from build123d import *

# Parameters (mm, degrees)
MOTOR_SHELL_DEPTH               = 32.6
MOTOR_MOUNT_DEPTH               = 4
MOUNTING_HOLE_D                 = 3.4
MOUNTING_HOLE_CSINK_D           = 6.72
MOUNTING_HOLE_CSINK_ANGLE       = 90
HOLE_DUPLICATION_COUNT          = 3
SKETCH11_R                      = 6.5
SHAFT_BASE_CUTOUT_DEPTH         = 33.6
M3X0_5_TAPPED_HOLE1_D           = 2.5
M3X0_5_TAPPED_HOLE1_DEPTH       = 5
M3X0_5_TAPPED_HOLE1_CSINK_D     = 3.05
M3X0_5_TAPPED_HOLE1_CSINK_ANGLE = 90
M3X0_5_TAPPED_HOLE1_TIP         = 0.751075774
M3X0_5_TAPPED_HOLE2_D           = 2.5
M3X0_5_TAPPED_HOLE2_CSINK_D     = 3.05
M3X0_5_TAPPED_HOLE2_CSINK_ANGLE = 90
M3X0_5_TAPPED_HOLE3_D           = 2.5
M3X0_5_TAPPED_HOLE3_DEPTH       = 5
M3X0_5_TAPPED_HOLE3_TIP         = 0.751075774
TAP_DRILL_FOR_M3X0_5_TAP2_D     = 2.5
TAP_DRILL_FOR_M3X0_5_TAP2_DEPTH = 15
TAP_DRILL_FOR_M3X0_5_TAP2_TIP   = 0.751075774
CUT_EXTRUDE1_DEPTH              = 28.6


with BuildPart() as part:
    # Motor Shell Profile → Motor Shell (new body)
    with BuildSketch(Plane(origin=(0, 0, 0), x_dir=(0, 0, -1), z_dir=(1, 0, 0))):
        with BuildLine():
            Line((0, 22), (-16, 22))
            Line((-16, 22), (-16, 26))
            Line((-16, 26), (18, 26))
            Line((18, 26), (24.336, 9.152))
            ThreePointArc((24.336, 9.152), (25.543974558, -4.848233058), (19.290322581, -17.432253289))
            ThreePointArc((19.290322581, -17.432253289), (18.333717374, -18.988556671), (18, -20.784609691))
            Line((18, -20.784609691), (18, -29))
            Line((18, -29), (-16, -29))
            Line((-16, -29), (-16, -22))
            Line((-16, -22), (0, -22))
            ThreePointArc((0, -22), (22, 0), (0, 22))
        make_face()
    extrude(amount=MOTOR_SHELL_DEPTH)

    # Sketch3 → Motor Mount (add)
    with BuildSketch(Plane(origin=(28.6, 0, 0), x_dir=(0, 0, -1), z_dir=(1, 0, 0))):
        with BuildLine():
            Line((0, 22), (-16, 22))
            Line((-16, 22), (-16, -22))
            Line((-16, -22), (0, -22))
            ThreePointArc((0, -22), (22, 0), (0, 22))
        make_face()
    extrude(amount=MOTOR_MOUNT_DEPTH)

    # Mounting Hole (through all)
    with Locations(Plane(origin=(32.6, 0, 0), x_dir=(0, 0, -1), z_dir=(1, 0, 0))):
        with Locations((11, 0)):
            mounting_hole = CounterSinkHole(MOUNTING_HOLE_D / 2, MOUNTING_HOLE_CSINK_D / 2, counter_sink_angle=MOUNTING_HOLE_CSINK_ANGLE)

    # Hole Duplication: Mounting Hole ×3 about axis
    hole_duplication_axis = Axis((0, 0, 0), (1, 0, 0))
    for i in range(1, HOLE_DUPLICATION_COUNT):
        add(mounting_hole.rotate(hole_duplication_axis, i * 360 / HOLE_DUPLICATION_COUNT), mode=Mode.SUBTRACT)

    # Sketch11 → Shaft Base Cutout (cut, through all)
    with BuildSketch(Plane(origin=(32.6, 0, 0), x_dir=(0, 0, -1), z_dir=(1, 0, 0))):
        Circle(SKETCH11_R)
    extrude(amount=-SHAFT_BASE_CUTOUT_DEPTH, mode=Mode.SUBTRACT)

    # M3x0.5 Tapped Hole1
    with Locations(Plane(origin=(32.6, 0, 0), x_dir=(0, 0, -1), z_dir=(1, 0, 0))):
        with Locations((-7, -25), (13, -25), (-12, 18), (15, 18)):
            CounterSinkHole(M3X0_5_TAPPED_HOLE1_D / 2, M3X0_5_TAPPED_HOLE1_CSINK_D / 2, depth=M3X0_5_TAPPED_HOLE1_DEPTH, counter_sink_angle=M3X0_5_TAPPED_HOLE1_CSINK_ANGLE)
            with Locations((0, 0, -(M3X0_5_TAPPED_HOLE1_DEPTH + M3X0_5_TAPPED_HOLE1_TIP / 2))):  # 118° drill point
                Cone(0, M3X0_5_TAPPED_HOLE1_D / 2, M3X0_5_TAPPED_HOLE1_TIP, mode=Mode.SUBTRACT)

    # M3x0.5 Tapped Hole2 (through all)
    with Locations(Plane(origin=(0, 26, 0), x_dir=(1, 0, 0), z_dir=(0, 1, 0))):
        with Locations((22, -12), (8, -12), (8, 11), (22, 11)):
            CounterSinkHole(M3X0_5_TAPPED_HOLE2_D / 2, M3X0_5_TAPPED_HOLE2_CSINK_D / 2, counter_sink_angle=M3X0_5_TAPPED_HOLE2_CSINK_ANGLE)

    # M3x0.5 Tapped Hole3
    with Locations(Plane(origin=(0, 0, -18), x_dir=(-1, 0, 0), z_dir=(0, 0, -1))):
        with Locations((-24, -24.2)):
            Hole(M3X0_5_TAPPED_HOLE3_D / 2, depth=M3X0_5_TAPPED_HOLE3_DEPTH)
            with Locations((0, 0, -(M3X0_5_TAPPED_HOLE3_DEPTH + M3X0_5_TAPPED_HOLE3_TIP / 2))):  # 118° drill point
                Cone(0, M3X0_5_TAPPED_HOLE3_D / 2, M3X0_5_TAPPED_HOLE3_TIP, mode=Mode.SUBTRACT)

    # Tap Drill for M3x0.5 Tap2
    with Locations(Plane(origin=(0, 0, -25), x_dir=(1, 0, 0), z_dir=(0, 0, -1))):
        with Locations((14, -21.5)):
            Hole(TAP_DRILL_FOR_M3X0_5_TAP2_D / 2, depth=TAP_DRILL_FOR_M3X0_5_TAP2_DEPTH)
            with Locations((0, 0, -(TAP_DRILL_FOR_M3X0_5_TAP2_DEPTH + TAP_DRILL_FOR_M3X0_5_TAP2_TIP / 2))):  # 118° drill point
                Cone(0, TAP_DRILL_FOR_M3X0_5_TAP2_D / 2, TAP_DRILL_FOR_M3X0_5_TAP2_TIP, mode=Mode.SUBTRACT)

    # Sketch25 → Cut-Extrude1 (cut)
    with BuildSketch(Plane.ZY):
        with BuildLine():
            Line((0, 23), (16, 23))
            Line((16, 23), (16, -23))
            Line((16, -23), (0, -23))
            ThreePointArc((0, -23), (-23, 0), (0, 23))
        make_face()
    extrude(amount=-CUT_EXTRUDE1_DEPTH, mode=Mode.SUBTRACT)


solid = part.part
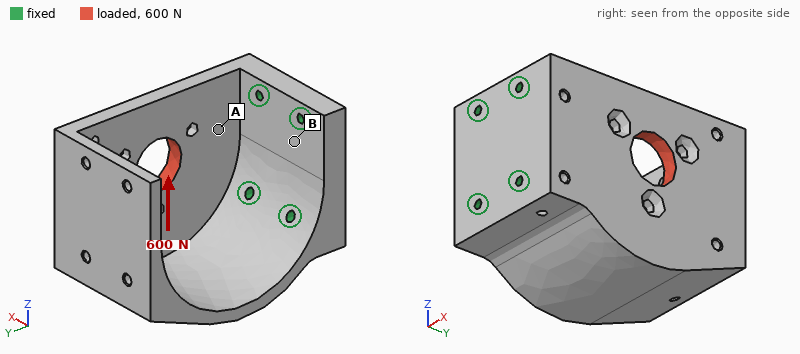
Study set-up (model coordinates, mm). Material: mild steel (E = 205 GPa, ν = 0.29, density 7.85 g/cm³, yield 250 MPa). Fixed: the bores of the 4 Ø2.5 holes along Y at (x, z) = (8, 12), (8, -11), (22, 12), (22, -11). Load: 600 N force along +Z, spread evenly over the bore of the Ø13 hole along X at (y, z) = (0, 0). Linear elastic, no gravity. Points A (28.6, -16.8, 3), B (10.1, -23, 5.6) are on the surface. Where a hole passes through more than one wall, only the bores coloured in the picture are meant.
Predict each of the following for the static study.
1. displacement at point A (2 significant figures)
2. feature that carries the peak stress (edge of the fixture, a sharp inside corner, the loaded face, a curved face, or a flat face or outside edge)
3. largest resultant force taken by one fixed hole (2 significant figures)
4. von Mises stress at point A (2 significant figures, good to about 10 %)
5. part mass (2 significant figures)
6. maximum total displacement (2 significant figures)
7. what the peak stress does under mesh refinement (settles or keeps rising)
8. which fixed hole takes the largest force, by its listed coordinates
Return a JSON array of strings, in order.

["2.7 µm", "edge of the fixture", "690 N", "14 MPa", "180 g", "16 µm", "keeps rising", "(22, -11)"]
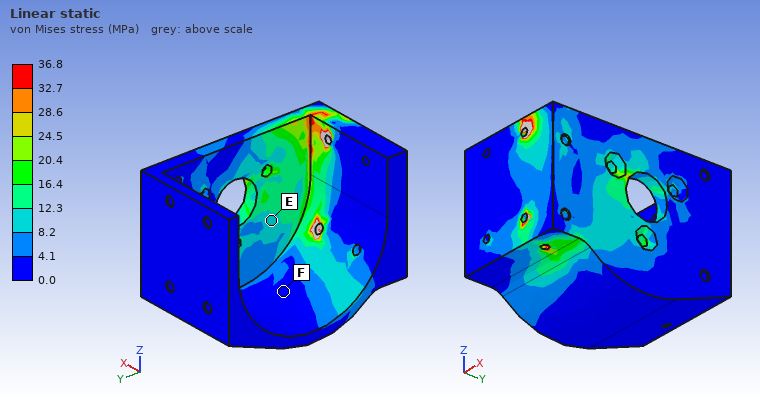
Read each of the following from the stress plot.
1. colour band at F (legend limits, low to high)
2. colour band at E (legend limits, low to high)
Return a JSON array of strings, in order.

["0.0 to 4.1 MPa", "8.2 to 12.3 MPa"]
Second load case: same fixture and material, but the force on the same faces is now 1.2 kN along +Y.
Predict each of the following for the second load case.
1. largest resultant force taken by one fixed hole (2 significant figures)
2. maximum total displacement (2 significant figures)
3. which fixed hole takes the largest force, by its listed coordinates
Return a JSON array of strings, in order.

["850 N", "13 µm", "(22, -11)"]
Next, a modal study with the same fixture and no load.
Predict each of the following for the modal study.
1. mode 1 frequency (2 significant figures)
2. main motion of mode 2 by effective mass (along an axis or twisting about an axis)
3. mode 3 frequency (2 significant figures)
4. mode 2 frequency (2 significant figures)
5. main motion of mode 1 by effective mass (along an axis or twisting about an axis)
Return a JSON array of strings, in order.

["1400 Hz", "along Z", "4300 Hz", "2500 Hz", "along X"]
